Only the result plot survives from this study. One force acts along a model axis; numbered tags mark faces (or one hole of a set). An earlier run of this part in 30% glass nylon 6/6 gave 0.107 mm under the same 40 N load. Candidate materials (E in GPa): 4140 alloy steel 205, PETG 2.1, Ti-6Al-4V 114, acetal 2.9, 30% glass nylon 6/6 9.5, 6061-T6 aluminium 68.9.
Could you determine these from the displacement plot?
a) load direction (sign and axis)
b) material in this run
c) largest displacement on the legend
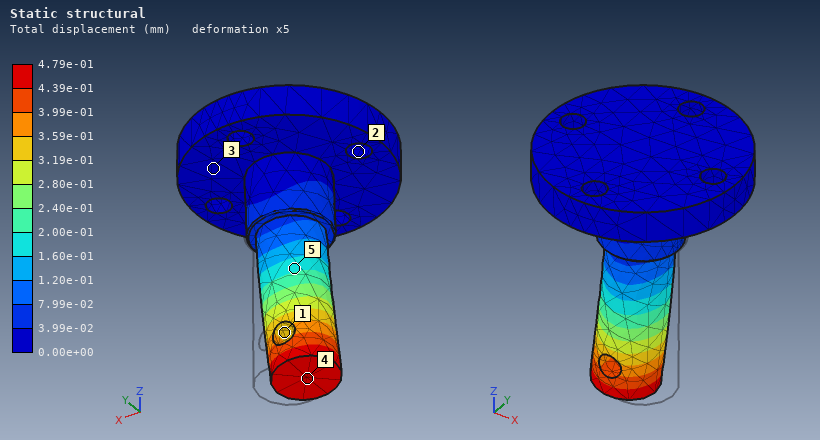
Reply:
-X
PETG
4.79e-01 mm
